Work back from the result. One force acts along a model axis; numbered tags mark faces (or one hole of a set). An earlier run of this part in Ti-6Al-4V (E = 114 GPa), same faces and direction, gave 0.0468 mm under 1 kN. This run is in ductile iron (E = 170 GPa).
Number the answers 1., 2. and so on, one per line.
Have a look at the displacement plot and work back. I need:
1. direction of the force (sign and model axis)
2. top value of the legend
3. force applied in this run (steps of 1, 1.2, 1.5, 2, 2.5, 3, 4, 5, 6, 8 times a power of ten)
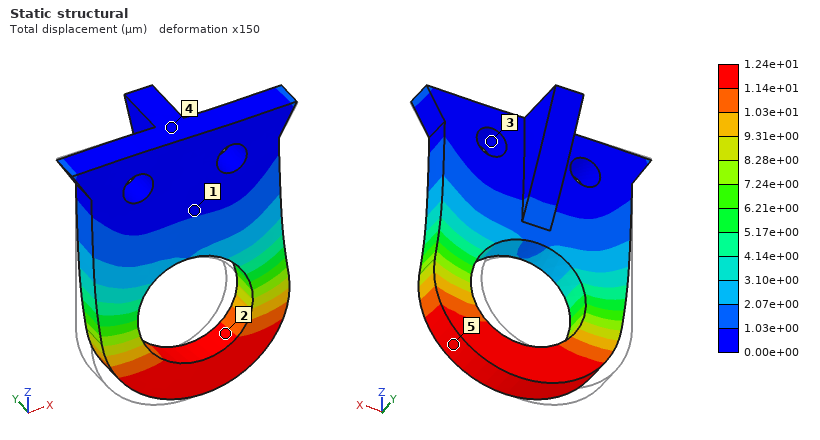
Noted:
1. +X
2. 1.24e+01 µm
3. 400 N
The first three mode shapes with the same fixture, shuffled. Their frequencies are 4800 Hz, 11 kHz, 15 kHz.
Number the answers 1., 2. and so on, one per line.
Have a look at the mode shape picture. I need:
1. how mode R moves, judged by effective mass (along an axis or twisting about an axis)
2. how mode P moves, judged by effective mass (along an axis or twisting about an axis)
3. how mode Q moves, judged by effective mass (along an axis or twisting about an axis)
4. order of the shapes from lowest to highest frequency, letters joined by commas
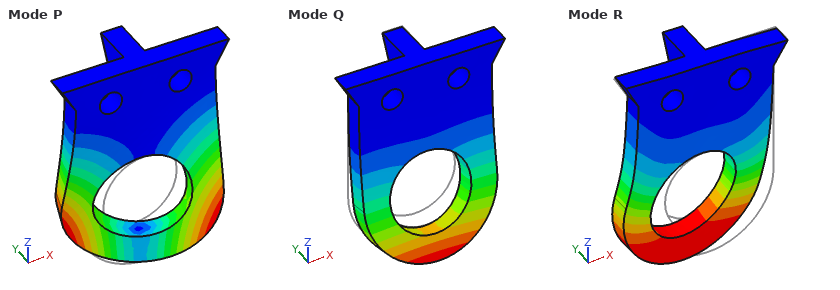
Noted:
1. along X
2. twisting about Z
3. along Y
4. Q, P, R
